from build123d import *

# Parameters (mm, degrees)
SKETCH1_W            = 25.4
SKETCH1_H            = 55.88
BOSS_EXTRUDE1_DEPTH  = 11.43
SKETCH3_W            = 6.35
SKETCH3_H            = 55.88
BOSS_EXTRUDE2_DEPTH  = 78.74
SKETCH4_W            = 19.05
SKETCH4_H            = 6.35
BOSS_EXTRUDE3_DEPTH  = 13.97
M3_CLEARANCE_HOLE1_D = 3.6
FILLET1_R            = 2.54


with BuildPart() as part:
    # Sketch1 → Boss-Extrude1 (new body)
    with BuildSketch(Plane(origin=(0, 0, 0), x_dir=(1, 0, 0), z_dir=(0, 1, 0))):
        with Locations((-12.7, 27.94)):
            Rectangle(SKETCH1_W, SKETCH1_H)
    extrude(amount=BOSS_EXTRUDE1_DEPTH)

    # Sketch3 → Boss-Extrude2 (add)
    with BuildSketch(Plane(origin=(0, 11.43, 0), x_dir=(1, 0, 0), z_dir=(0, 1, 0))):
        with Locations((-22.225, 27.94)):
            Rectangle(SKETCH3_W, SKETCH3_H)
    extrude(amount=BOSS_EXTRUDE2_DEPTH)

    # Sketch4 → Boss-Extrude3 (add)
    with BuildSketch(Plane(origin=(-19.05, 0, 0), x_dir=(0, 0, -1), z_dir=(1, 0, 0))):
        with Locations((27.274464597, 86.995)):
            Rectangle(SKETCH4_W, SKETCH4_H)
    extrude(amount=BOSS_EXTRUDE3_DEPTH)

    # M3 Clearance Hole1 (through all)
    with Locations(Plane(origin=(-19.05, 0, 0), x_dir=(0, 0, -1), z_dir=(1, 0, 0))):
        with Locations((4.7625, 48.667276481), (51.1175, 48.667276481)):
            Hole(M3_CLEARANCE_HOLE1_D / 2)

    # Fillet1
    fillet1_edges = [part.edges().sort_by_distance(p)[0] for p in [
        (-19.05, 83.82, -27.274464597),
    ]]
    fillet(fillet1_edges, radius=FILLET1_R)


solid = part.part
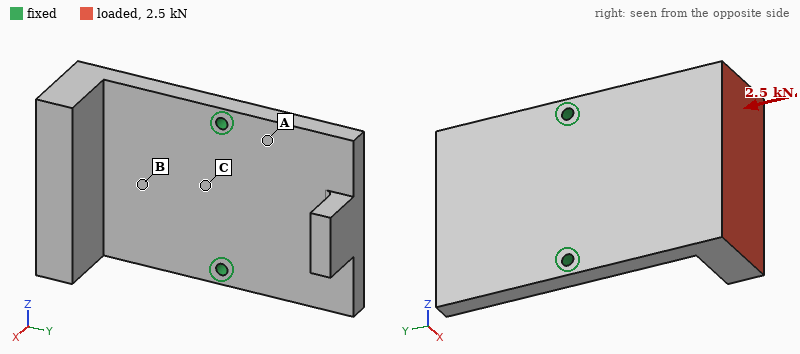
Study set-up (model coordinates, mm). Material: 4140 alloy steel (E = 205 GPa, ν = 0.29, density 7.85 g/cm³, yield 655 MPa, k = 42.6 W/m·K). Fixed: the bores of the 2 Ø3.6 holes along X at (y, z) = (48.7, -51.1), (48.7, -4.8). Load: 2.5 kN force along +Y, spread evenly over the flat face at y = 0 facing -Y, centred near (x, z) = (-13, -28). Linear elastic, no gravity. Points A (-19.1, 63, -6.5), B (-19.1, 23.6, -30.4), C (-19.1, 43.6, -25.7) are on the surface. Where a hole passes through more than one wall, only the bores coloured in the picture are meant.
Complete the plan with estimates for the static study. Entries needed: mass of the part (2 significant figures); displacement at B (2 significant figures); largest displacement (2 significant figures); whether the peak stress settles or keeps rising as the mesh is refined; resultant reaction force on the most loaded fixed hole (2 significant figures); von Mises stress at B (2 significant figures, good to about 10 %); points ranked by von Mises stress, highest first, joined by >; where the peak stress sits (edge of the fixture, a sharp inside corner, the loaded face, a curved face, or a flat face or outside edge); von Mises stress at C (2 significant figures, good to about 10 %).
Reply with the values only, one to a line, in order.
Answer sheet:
360 g
0.044 mm
0.16 mm
keeps rising
1.3 kN
64 MPa
B > C > A
edge of the fixture
44 MPa
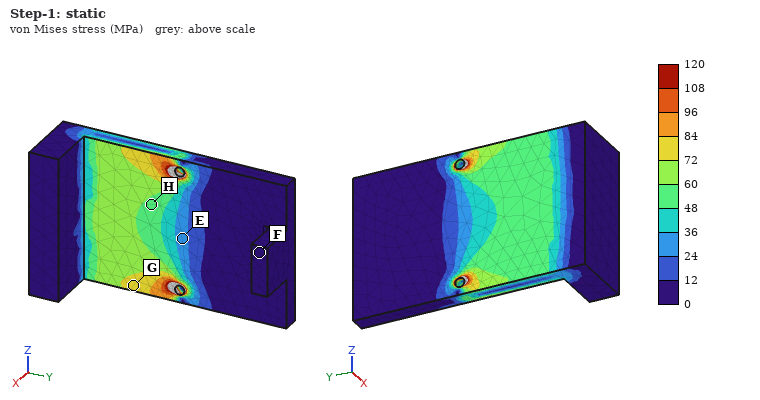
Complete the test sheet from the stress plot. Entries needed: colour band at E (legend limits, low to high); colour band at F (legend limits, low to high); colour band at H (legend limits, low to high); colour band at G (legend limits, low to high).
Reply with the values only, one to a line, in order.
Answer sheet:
24 to 36 MPa
0 to 12 MPa
48 to 60 MPa
72 to 84 MPa
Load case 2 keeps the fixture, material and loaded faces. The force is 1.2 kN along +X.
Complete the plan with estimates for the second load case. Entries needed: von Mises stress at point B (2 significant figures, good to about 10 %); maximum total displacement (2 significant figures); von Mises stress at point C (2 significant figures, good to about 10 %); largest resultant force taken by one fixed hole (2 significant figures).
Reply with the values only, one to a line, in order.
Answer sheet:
72 MPa
0.28 mm
83 MPa
600 N
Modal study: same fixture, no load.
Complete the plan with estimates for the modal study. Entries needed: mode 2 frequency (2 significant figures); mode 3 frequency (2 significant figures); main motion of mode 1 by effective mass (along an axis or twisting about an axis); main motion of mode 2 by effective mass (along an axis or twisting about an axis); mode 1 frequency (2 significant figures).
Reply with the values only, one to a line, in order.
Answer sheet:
2200 Hz
2800 Hz
along X
along X
1000 Hz
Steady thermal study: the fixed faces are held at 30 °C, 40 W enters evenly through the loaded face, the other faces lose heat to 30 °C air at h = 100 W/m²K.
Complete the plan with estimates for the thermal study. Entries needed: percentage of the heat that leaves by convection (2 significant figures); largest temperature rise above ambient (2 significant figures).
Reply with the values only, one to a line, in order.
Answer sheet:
72 %
62 K
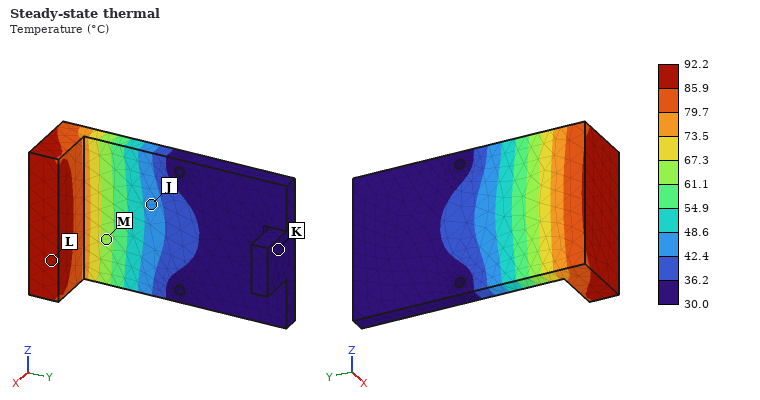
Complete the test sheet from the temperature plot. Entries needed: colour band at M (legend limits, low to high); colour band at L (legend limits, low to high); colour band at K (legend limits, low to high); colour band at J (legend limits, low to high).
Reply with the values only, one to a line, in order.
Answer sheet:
61.1 to 67.3 °C
85.9 to 92.2 °C
30.0 to 36.2 °C
42.4 to 48.6 °C
